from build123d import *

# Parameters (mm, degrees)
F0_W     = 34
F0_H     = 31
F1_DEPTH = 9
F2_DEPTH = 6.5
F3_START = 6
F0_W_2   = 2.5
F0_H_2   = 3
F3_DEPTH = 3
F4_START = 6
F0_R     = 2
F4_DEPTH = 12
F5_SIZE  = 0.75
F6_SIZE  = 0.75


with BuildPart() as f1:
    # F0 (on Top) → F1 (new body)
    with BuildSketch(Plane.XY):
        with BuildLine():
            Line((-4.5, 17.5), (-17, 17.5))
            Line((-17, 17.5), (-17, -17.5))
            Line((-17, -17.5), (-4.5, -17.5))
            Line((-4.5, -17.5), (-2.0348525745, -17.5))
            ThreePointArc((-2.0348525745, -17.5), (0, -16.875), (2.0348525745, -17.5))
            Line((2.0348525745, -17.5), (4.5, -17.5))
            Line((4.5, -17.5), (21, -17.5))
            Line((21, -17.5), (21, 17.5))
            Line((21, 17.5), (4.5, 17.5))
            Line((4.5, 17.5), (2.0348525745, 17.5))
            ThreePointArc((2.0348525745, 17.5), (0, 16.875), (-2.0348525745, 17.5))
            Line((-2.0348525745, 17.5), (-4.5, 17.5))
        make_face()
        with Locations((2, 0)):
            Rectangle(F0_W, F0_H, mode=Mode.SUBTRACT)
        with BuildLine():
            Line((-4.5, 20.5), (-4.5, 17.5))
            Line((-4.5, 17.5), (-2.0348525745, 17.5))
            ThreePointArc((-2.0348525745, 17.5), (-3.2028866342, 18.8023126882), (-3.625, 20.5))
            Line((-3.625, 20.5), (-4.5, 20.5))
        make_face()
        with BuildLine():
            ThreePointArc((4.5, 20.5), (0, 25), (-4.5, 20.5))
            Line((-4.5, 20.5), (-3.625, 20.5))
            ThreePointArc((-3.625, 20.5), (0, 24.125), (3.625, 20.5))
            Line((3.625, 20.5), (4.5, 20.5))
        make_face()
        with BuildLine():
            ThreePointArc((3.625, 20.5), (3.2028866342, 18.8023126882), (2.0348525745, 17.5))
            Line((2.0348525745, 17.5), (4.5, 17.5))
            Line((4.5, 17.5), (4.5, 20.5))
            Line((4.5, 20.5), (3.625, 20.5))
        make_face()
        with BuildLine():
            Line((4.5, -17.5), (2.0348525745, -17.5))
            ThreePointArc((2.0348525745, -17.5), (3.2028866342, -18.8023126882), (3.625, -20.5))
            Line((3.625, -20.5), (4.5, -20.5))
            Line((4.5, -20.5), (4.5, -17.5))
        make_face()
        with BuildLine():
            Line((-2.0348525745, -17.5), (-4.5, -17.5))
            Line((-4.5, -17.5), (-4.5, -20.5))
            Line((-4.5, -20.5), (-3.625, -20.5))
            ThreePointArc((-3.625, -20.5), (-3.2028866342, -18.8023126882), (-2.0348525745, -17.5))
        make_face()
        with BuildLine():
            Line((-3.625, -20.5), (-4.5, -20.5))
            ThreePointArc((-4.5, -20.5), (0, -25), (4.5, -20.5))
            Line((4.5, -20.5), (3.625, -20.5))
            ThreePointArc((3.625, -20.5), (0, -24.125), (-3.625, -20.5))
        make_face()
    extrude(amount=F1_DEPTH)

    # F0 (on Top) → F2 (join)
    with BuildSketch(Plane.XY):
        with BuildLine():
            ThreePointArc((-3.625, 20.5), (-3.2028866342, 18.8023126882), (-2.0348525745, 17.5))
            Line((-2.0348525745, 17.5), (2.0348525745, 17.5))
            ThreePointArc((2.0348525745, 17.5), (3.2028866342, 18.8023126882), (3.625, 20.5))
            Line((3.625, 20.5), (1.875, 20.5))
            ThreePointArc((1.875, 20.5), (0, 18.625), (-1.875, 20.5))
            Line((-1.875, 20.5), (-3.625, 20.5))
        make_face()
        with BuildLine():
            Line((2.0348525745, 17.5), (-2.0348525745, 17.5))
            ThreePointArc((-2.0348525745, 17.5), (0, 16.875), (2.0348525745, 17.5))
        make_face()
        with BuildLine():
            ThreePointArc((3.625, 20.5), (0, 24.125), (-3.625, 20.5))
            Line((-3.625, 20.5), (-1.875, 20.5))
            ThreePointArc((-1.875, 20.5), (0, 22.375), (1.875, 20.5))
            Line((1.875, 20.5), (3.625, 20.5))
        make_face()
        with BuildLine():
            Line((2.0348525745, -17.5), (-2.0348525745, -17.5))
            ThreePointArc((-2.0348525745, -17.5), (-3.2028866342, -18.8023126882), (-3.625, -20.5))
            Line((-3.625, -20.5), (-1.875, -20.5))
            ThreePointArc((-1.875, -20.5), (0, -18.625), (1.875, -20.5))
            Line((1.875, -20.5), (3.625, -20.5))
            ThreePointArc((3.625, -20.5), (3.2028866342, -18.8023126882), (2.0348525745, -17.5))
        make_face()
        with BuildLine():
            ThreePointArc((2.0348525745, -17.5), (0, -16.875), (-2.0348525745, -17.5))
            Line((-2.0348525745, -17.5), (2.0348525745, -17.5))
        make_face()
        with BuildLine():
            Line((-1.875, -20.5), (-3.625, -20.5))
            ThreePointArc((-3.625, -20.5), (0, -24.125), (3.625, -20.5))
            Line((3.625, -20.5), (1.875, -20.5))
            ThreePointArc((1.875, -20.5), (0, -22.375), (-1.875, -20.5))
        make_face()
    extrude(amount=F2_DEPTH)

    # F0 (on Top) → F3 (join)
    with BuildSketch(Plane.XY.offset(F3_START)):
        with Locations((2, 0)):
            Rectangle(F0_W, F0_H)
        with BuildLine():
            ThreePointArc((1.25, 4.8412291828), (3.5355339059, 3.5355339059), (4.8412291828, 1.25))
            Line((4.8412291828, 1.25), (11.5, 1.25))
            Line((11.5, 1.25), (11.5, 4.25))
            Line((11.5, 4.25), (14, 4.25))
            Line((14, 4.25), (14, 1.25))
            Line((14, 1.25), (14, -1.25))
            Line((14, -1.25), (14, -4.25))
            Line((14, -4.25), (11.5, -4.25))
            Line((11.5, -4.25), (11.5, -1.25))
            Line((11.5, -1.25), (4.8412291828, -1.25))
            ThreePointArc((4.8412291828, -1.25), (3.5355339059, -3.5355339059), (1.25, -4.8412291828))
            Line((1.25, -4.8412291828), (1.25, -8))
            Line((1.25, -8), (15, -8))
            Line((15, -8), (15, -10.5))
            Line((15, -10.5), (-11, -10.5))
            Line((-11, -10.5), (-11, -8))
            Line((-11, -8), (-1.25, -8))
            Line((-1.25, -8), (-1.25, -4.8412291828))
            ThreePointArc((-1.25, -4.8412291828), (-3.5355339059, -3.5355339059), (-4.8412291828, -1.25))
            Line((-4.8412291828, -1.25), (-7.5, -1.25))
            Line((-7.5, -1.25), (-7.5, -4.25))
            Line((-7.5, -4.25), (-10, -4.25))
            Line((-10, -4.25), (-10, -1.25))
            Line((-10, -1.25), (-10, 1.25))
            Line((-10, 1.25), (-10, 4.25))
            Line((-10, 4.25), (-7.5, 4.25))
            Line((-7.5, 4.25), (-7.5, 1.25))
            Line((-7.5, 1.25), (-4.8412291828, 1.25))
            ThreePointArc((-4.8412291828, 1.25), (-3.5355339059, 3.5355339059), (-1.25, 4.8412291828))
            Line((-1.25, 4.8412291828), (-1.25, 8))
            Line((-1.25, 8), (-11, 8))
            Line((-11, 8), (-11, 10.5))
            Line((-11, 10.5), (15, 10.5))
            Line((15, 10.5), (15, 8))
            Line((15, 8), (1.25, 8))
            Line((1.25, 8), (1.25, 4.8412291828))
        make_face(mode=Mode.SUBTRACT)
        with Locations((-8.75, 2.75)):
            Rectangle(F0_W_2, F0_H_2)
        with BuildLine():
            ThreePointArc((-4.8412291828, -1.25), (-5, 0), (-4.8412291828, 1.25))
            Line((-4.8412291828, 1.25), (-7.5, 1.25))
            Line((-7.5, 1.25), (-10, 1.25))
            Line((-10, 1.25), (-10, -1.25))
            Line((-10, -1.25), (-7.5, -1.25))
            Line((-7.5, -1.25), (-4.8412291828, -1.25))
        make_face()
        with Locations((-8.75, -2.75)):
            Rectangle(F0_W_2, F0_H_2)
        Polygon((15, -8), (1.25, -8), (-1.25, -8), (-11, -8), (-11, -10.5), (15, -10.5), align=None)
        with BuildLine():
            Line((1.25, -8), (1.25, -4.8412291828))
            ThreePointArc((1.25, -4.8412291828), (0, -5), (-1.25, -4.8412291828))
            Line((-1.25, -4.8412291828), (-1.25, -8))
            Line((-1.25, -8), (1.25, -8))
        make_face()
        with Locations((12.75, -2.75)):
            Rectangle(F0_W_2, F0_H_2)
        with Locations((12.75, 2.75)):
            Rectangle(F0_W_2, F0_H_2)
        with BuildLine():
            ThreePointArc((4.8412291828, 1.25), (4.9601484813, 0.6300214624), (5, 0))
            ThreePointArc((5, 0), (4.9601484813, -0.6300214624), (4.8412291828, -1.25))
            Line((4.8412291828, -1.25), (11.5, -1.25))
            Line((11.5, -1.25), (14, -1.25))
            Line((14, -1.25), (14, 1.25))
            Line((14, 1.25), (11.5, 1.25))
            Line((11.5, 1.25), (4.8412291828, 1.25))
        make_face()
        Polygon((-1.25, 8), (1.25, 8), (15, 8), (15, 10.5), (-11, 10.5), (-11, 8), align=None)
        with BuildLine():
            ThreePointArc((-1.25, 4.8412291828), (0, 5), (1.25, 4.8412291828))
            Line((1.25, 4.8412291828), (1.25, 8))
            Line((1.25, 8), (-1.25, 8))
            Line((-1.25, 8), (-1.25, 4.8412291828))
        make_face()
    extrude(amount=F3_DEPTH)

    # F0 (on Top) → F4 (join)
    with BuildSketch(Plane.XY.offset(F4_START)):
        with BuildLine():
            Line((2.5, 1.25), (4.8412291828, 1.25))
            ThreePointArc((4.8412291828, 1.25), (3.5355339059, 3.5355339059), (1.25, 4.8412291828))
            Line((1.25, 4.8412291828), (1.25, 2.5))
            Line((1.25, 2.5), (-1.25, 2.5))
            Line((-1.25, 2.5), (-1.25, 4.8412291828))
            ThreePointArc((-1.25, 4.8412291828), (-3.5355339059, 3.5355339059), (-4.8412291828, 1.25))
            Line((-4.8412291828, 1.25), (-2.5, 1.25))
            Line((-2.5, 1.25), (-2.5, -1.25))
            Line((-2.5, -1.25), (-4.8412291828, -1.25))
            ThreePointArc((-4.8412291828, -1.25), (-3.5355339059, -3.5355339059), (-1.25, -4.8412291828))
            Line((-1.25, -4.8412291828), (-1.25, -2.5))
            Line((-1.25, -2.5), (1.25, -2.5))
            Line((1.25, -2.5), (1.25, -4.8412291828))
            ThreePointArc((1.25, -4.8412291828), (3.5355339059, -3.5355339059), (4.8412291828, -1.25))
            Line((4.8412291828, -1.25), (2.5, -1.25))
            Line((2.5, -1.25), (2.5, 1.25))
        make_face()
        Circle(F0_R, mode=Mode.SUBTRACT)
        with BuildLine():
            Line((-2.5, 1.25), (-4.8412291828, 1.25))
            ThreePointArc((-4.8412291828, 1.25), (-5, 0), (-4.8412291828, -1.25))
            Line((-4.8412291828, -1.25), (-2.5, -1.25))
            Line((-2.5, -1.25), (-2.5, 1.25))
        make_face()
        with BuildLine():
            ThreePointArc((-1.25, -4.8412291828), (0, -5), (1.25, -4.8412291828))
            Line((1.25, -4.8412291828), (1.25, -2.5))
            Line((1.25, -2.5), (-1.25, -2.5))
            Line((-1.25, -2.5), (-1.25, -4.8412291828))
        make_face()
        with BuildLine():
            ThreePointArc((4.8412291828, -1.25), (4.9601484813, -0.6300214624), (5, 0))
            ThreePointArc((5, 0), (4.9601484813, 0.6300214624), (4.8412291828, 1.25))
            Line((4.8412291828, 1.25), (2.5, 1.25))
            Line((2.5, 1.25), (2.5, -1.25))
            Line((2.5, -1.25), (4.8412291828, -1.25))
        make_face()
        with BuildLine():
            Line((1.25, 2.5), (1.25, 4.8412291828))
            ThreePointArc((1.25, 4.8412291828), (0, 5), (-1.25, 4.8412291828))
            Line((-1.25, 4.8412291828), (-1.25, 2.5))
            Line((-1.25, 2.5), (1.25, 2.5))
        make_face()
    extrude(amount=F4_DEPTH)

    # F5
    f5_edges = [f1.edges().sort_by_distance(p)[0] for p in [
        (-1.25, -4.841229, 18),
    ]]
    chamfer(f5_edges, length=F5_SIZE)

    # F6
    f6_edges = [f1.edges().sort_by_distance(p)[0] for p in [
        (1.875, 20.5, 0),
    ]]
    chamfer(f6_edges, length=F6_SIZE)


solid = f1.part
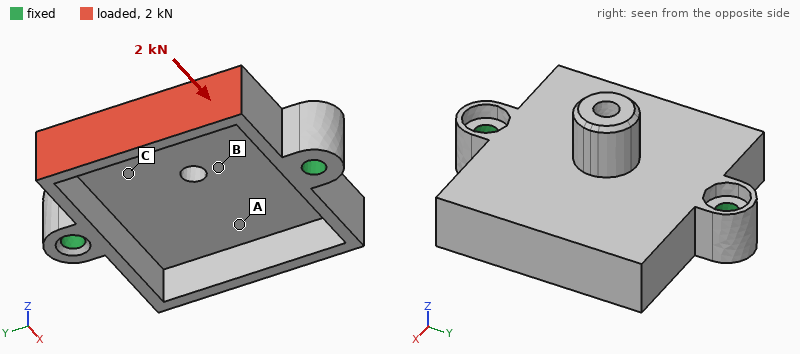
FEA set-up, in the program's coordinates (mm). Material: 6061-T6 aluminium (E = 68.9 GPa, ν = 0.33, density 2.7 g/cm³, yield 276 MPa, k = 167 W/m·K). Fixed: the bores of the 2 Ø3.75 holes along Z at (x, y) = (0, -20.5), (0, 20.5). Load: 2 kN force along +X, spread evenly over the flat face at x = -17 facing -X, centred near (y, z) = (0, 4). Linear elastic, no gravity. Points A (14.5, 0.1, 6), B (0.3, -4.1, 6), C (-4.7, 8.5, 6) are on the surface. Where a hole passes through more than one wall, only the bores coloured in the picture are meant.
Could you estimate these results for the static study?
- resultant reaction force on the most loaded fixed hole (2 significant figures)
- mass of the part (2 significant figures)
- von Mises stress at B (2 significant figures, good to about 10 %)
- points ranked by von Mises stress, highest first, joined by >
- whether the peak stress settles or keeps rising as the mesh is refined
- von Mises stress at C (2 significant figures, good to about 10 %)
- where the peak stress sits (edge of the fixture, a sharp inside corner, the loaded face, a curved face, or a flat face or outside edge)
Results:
1.0 kN
19 g
19 MPa
C > B > A
keeps rising
31 MPa
edge of the fixture
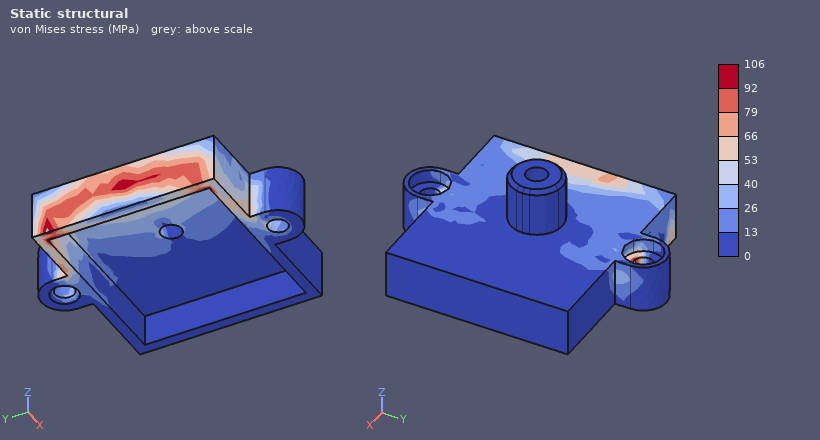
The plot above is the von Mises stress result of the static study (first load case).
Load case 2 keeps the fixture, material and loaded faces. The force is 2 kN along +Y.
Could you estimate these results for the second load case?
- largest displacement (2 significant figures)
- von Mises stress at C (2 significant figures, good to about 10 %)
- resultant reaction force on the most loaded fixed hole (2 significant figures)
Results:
72 µm
51 MPa
1.3 kN
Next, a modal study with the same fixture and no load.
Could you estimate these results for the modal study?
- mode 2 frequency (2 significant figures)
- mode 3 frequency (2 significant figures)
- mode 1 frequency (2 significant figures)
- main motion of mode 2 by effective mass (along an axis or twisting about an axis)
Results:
9300 Hz
11 kHz
6200 Hz
along Z
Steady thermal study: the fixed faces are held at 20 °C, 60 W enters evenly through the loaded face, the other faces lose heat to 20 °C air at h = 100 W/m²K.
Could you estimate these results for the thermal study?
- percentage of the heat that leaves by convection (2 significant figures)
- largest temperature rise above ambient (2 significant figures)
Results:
19 %
68 K
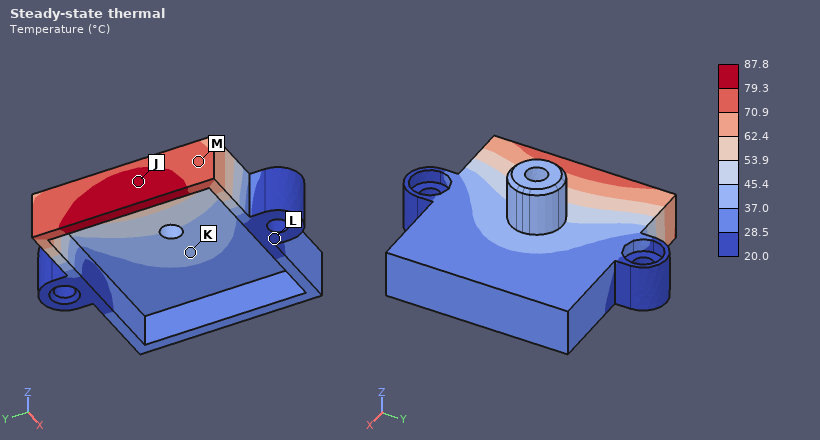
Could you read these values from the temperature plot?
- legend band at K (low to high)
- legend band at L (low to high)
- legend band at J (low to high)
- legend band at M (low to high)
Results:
37.0 to 45.4 °C
20.0 to 28.5 °C
79.3 to 87.8 °C
70.9 to 79.3 °C
